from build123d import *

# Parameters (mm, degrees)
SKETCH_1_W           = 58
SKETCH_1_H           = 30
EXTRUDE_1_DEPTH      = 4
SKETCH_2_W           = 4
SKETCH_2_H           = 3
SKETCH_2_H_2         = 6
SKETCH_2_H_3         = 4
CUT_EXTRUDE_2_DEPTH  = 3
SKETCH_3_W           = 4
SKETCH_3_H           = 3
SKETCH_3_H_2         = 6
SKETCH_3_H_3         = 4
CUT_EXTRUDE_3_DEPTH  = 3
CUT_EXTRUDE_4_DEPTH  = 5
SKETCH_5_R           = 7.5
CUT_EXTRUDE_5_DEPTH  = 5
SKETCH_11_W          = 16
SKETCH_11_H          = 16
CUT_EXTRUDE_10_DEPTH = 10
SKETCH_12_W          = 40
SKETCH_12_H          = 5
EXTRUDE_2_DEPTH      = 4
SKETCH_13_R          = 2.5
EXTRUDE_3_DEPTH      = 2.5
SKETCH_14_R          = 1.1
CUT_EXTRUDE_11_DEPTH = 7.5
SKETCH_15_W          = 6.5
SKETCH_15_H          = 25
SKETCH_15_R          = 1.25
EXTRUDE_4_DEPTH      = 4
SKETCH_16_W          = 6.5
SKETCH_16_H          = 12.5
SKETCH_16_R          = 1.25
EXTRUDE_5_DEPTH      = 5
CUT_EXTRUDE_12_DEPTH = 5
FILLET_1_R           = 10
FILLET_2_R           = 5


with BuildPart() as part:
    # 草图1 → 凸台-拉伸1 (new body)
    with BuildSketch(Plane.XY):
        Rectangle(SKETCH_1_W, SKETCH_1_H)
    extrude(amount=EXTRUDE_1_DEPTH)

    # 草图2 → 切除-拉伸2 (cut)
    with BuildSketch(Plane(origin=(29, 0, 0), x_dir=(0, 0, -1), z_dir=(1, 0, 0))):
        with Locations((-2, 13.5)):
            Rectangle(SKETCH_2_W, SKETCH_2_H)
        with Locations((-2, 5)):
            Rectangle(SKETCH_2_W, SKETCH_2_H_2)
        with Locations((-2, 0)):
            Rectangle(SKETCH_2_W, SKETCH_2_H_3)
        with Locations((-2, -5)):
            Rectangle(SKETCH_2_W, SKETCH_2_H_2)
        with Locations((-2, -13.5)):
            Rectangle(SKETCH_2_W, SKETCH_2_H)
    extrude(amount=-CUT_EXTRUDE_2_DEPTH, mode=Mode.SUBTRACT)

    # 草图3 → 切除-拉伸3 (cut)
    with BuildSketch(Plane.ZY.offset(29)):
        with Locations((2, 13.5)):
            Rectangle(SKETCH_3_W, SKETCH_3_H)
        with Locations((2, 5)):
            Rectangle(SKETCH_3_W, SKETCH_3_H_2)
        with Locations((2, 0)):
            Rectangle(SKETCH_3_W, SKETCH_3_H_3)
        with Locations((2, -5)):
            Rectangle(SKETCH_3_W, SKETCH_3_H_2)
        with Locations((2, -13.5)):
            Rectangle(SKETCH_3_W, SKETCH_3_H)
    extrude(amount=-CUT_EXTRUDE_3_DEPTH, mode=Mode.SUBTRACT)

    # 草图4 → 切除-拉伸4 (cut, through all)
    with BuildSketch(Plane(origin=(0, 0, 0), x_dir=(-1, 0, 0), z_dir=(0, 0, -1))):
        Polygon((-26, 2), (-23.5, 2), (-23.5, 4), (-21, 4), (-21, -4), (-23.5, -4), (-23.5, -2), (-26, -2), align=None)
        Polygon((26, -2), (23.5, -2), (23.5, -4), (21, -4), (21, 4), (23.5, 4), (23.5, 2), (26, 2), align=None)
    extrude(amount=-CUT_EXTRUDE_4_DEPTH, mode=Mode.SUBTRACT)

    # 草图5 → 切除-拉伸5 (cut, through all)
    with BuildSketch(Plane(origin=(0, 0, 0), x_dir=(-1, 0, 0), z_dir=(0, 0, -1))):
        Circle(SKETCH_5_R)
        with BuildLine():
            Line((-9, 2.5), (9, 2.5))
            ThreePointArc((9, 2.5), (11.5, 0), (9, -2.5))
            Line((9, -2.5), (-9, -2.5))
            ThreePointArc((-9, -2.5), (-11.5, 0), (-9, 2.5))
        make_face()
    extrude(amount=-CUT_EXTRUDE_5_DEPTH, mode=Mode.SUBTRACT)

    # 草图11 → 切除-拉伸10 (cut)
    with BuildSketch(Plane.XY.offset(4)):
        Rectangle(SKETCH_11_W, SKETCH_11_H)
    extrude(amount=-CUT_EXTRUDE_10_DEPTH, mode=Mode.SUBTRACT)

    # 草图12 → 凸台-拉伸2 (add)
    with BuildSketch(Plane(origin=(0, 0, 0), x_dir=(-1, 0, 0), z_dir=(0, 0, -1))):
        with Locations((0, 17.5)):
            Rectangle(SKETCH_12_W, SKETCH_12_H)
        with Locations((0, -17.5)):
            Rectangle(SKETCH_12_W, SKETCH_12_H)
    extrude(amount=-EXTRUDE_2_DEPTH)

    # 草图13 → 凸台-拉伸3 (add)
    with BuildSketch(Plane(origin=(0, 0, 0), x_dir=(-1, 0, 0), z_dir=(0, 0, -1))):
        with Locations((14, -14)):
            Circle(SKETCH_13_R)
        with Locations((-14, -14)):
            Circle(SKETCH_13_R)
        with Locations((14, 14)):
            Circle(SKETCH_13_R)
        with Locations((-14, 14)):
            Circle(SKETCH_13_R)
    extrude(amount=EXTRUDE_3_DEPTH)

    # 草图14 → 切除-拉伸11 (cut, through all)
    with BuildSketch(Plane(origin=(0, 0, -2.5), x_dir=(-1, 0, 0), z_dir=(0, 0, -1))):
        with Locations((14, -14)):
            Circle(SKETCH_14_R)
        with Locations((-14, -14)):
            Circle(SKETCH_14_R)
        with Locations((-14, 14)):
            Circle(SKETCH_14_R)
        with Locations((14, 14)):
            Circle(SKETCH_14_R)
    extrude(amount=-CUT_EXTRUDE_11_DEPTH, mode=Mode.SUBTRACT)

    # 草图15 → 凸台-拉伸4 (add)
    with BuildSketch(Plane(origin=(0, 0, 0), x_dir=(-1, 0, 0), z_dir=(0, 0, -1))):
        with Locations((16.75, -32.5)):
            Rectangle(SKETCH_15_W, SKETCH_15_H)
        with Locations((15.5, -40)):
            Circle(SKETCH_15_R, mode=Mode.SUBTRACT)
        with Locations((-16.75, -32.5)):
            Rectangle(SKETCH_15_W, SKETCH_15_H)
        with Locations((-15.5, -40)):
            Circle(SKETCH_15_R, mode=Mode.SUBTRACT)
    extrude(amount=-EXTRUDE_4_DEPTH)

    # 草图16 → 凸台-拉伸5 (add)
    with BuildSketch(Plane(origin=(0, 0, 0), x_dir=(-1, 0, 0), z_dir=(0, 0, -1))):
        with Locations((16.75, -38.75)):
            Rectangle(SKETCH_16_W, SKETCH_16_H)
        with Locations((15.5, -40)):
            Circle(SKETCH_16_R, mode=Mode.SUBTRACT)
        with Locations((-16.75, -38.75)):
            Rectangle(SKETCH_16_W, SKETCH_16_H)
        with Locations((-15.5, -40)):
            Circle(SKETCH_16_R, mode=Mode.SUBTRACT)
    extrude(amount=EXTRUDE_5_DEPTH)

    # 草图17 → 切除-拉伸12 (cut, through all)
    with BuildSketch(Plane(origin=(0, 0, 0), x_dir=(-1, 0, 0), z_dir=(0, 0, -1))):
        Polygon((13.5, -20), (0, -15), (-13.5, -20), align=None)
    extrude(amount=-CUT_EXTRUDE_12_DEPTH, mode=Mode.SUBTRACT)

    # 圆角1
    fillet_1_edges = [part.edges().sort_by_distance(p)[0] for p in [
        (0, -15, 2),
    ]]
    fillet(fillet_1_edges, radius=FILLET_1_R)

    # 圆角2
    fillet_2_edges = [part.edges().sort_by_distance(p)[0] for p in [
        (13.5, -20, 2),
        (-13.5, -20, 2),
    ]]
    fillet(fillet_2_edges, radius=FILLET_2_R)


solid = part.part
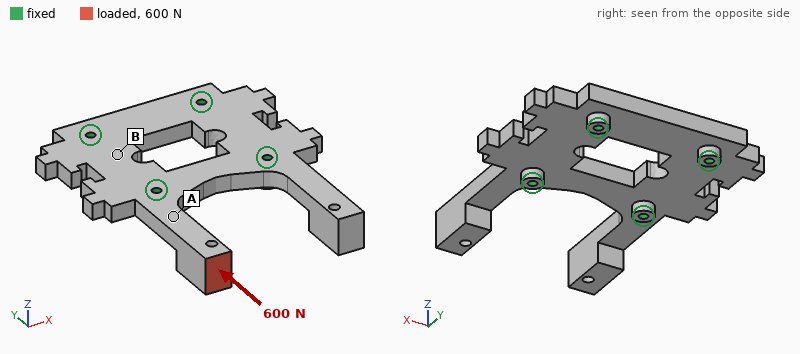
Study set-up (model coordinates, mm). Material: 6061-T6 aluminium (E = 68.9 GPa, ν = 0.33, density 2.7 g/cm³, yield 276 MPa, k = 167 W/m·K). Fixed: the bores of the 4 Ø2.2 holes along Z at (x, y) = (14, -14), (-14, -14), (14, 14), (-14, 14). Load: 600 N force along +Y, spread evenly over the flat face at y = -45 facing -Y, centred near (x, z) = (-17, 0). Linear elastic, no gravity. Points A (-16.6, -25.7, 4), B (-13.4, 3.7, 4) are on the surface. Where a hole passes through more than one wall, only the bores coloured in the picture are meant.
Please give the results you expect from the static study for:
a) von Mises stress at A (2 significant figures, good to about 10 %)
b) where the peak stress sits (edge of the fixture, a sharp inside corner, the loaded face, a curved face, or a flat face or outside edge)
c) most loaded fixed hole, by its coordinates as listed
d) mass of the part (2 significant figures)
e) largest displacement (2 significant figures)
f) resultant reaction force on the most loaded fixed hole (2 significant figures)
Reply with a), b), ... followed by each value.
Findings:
a) 63 MPa
b) a curved face
c) (-14, -14)
d) 23 g
e) 0.24 mm
f) 540 N
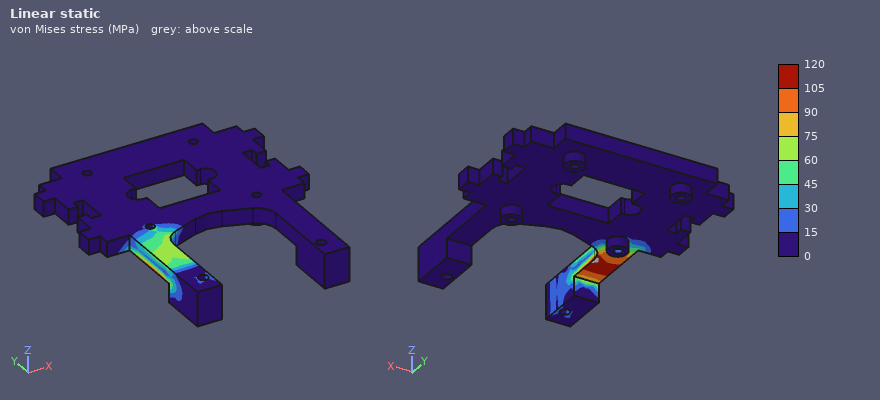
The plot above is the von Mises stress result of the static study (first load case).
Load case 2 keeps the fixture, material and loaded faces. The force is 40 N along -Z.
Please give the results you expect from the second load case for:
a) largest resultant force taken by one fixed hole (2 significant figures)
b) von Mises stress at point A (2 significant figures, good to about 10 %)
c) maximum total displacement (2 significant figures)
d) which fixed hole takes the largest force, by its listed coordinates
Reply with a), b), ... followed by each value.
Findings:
a) 52 N
b) 44 MPa
c) 0.14 mm
d) (-14, -14)
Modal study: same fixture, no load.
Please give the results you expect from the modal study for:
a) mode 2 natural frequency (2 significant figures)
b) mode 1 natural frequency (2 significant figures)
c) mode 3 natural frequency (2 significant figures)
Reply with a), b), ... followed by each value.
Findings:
a) 2600 Hz
b) 2600 Hz
c) 4400 Hz
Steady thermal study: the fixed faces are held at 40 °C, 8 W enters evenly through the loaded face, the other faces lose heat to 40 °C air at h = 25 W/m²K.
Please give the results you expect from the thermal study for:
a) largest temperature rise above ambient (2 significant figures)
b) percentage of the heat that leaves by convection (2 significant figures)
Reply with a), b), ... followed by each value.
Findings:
a) 43 K
b) 7.5 %
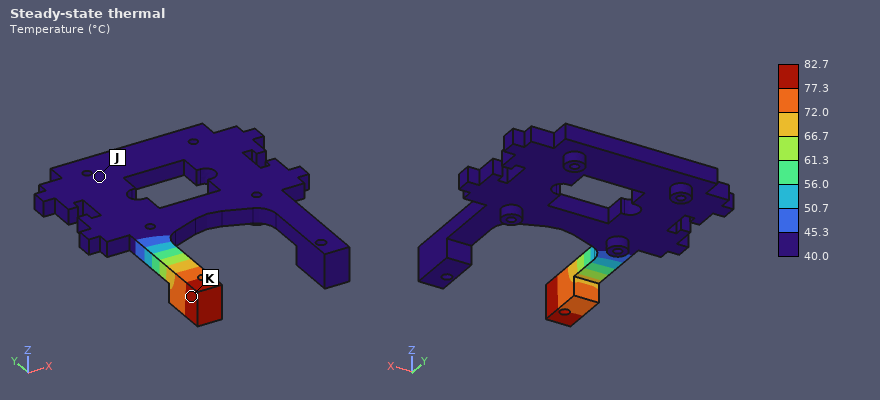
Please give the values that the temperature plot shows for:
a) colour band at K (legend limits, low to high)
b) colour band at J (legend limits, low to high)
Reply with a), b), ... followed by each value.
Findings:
a) 77.3 to 82.7 °C
b) 40.0 to 45.3 °C
